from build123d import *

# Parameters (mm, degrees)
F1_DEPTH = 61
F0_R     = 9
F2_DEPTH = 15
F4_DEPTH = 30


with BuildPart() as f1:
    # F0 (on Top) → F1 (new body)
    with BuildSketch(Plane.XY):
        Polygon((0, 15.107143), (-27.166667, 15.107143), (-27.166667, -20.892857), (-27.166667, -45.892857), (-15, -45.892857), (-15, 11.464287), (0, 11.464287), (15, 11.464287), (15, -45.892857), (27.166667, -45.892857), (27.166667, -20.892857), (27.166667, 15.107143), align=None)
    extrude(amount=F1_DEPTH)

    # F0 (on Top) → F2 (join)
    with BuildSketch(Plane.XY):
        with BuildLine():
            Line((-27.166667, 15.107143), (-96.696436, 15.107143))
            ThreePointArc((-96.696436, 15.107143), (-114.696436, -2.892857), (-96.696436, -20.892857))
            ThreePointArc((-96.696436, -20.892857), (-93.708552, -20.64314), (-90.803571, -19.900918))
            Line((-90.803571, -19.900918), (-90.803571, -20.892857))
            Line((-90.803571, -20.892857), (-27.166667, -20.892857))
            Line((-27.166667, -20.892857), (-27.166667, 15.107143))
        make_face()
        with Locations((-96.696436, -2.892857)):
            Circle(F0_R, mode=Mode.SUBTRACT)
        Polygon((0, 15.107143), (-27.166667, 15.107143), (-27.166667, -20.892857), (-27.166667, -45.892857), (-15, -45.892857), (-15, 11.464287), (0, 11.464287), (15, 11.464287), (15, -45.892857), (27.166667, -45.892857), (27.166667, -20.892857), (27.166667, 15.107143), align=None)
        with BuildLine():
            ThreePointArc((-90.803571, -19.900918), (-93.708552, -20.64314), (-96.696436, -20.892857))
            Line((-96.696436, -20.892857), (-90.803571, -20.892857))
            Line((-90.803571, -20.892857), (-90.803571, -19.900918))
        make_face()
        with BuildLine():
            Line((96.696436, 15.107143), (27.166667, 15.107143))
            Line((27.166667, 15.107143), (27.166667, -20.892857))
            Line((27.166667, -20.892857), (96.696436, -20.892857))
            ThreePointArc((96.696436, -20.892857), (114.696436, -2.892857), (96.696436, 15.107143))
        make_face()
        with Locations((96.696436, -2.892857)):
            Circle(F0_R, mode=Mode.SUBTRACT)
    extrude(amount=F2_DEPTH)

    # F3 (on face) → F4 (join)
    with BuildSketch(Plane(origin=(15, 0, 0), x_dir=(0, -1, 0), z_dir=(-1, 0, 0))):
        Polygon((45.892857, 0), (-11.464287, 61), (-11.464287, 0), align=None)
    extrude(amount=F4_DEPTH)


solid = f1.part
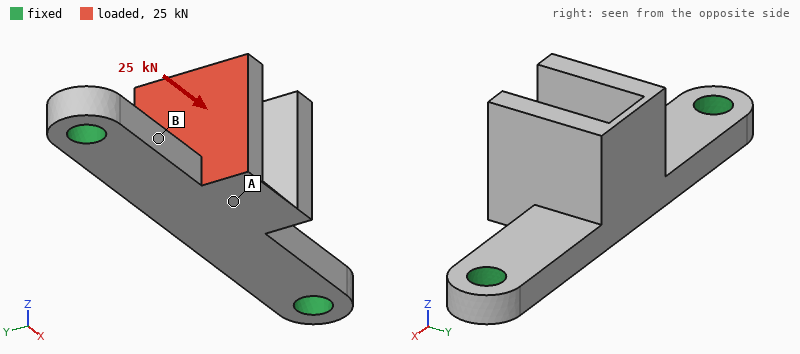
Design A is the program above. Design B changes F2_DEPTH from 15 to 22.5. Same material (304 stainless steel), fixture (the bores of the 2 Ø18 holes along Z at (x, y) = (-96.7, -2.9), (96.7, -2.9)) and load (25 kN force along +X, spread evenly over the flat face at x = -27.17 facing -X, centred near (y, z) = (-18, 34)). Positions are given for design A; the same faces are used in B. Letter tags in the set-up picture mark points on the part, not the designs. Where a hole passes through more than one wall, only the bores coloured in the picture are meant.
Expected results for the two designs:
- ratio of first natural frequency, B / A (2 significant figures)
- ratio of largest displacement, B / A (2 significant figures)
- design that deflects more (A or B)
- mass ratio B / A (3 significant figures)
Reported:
1.6
0.70
A
1.18
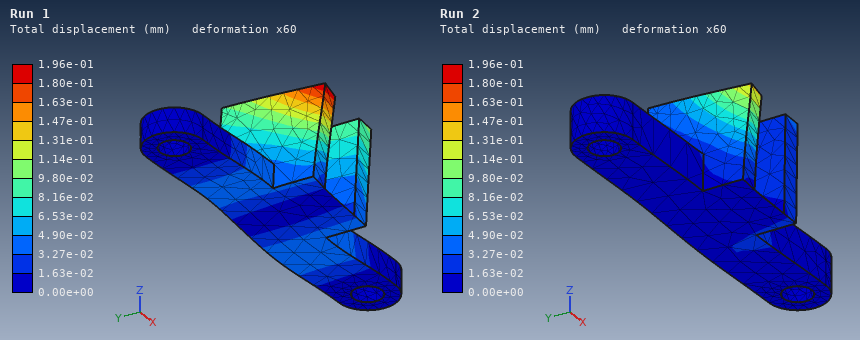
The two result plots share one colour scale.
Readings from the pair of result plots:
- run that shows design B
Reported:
Run 2
